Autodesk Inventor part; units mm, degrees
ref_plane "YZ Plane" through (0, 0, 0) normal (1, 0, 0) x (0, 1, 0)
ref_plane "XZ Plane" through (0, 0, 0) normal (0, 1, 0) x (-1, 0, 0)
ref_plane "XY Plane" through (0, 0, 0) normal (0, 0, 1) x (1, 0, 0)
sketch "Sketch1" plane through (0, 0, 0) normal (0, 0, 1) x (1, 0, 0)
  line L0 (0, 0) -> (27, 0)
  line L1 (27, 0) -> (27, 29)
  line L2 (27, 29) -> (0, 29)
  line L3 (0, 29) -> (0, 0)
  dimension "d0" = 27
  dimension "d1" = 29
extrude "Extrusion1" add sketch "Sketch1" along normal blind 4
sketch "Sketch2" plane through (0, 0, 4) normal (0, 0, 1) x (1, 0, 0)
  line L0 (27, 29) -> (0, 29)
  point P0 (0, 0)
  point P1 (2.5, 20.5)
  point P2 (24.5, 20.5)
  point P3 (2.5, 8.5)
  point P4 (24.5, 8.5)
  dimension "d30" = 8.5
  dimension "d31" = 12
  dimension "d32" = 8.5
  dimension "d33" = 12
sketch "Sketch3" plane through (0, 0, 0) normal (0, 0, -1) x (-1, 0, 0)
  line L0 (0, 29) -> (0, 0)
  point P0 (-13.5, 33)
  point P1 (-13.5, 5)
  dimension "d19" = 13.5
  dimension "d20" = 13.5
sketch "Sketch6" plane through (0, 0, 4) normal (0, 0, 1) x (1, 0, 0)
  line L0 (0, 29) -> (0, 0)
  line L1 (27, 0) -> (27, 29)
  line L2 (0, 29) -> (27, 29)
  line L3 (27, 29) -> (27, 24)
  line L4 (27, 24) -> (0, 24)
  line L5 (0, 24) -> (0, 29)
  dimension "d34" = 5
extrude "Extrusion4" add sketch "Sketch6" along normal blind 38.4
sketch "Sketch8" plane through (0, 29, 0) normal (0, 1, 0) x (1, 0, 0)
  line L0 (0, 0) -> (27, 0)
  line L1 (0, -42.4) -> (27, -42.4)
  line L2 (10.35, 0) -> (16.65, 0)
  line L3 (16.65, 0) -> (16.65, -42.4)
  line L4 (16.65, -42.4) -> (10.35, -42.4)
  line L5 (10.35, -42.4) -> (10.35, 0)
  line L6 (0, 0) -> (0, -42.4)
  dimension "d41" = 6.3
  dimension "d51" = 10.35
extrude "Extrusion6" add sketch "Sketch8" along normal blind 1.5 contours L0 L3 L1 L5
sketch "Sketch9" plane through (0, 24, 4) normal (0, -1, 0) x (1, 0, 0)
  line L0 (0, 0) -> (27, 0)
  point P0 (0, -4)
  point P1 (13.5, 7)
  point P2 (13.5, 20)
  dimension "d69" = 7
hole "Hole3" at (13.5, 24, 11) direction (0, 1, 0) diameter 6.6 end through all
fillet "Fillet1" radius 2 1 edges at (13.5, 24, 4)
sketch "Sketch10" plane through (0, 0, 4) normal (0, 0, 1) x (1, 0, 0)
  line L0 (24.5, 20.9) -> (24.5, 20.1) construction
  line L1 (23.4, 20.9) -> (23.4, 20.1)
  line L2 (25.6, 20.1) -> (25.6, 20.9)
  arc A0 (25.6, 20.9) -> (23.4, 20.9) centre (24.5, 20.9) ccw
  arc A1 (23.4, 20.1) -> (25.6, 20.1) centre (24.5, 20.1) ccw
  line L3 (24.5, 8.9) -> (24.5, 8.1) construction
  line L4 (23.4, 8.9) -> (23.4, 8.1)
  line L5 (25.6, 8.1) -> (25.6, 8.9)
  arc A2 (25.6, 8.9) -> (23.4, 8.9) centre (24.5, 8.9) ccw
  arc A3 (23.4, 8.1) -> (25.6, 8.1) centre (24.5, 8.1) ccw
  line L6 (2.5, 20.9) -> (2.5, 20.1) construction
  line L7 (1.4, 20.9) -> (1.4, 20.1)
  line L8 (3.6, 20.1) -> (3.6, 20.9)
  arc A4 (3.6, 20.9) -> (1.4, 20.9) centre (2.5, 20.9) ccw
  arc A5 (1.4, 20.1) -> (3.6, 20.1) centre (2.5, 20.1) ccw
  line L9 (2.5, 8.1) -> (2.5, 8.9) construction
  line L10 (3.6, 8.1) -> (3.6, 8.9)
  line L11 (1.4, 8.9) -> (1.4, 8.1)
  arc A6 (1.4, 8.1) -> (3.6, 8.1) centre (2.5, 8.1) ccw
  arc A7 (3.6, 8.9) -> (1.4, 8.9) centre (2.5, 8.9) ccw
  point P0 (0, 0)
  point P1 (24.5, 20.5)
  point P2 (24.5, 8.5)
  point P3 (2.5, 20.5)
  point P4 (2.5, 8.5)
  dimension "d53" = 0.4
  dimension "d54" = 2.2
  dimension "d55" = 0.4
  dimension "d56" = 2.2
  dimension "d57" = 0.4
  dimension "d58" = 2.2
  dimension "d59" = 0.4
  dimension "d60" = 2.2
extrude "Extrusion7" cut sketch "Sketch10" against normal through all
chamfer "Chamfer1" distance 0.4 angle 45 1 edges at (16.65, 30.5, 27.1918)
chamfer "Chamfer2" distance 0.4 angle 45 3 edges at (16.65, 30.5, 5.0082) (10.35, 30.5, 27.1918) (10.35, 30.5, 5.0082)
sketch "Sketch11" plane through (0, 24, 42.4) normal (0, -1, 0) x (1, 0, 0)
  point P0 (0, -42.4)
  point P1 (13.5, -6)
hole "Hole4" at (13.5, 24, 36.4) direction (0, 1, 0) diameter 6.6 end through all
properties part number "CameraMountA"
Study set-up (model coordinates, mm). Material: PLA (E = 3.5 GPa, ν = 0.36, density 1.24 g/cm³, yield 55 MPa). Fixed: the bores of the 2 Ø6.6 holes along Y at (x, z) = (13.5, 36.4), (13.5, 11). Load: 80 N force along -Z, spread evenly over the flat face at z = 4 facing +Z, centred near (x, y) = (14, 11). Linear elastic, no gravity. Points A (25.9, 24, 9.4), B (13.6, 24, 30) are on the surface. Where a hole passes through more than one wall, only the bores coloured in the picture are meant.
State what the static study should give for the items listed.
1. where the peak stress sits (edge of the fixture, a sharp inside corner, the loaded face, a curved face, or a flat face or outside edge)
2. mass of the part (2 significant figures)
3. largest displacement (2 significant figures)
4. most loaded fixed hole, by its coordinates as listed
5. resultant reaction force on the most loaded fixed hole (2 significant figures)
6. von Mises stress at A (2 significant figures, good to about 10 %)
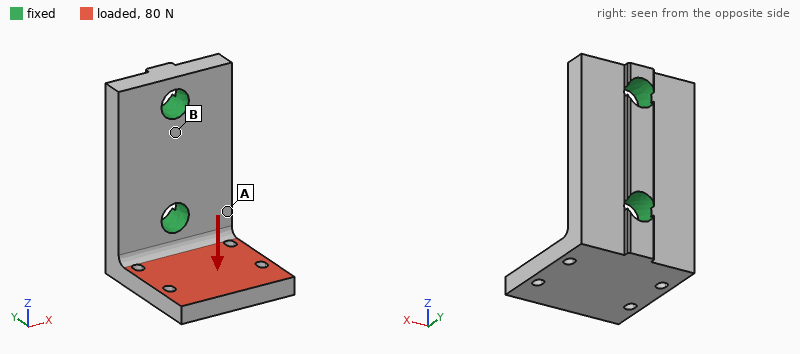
a sharp inside corner
10 g
0.52 mm
(13.5, 11)
70 N
4.4 MPa
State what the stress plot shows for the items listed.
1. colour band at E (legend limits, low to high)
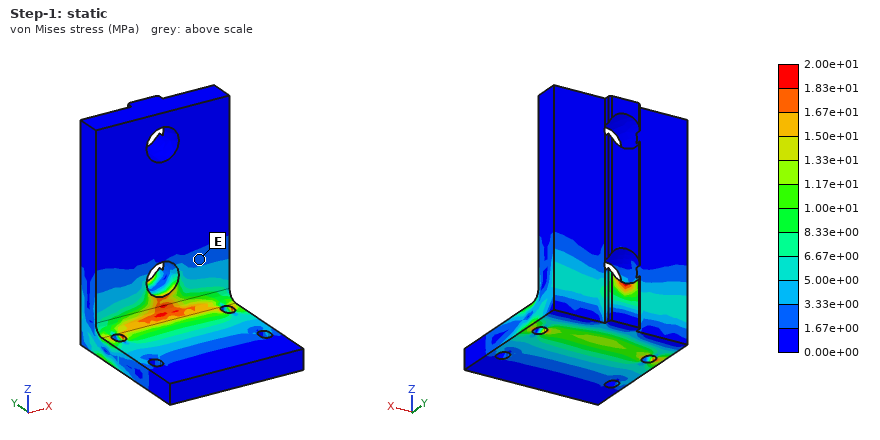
1.67e+00 to 3.33e+00 MPa
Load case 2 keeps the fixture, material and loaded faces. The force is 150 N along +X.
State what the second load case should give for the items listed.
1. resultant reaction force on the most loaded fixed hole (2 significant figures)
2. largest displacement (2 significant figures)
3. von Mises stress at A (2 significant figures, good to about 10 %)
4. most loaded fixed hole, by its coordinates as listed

170 N
0.35 mm
4.8 MPa
(13.5, 11)
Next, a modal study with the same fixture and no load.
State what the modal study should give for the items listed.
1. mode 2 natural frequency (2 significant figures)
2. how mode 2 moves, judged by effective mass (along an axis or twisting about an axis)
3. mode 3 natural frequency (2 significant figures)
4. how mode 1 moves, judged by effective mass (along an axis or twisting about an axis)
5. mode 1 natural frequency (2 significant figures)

2300 Hz
along X
3500 Hz
along Z
1400 Hz
